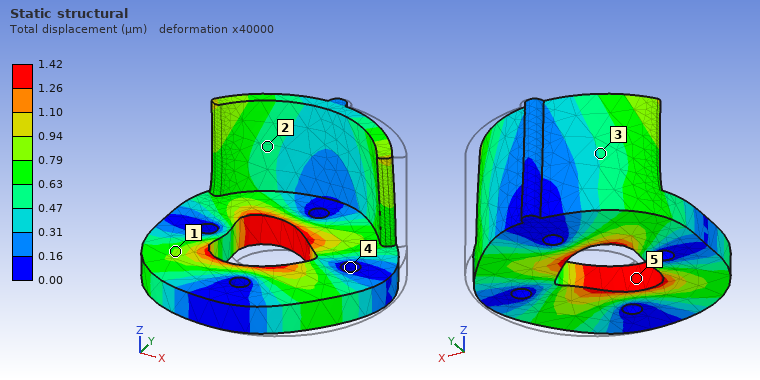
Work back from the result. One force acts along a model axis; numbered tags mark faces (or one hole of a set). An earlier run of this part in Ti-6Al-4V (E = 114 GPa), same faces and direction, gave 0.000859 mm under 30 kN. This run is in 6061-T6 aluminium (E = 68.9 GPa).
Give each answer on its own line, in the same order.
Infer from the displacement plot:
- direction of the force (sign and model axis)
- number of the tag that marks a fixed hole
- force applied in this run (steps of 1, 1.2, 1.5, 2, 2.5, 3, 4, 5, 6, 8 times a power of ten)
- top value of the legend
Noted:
-X
4
30 kN
1.42 µm
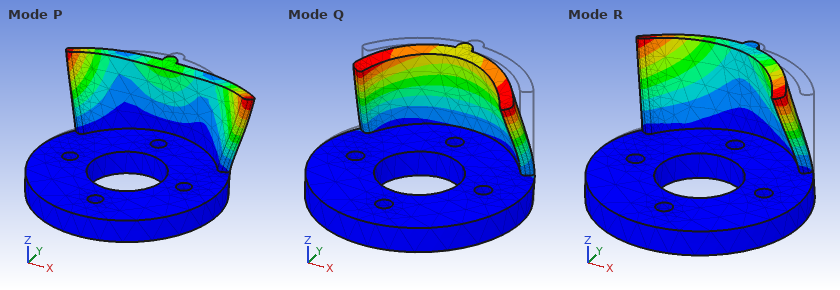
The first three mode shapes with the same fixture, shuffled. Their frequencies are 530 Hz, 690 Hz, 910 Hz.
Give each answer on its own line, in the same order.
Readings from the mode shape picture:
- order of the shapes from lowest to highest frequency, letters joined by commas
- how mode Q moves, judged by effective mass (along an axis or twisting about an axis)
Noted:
R, Q, P
along Y
